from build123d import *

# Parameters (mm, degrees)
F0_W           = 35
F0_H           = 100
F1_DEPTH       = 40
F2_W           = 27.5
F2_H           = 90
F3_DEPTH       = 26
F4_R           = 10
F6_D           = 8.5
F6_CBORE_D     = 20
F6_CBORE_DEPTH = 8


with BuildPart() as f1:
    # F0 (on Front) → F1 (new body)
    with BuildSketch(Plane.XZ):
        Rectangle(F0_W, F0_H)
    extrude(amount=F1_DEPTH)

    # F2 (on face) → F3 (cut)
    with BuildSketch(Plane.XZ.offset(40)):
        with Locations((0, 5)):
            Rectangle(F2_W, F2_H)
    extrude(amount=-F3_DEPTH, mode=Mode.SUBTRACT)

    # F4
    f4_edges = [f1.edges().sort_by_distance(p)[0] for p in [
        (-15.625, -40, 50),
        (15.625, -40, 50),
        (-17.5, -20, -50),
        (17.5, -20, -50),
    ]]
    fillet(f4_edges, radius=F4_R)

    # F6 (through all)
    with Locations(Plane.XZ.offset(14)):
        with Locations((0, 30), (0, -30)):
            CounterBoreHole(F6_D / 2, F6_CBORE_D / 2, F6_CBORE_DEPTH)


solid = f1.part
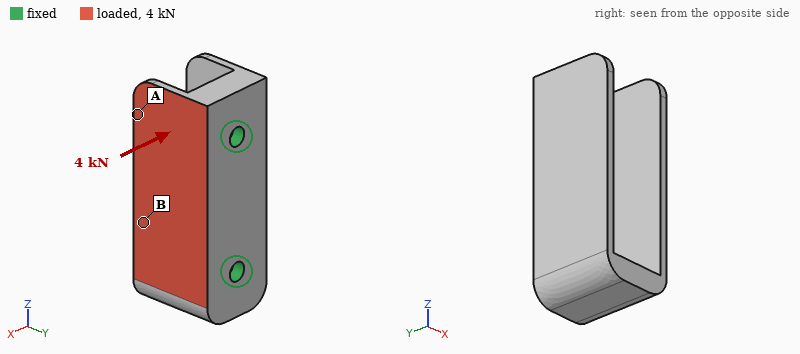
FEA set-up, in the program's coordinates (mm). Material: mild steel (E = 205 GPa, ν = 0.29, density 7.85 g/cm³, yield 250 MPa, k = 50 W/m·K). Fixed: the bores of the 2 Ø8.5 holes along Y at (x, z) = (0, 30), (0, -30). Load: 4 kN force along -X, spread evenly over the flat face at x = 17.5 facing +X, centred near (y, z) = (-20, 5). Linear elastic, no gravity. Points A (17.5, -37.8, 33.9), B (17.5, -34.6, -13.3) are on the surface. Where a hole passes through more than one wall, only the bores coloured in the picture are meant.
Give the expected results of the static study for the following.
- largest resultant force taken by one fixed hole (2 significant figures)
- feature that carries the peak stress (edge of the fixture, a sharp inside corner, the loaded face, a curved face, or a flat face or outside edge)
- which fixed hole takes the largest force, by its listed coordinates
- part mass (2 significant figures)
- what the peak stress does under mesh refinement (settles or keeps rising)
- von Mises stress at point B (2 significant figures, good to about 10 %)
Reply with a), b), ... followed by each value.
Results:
a) 2.3 kN
b) edge of the fixture
c) (0, 30)
d) 530 g
e) keeps rising
f) 47 MPa
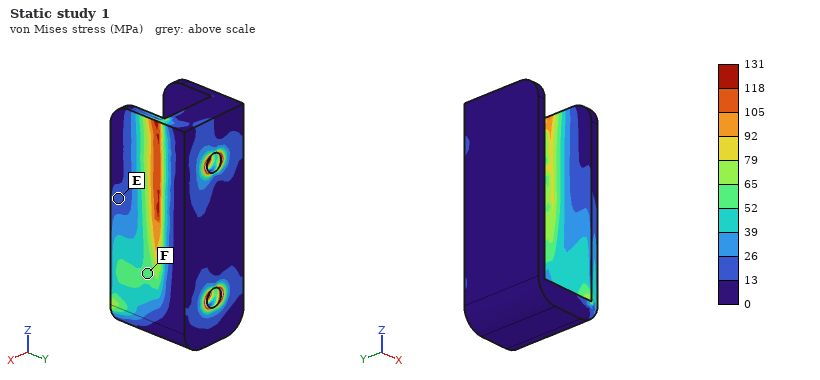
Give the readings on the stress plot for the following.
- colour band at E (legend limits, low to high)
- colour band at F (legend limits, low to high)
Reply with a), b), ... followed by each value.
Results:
a) 13 to 26 MPa
b) 52 to 65 MPa
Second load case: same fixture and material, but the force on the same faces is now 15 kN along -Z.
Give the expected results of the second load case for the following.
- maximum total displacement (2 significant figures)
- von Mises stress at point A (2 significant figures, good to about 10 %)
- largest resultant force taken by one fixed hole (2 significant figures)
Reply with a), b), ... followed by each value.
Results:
a) 29 µm
b) 28 MPa
c) 9.5 kN
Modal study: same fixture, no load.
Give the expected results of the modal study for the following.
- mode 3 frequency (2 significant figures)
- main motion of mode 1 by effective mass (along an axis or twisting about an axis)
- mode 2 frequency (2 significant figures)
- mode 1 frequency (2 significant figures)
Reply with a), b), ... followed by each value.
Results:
a) 4400 Hz
b) along X
c) 4300 Hz
d) 3100 Hz
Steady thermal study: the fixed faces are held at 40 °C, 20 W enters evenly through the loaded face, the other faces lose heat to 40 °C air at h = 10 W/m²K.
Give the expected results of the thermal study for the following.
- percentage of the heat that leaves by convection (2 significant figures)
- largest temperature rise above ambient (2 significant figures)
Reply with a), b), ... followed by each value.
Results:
a) 6.9 %
b) 21 K
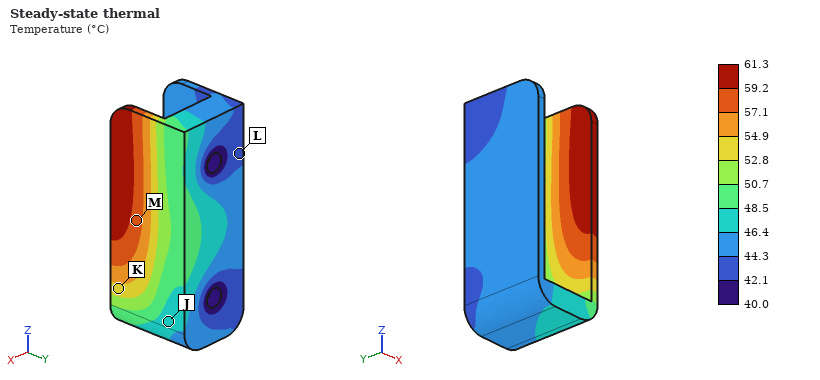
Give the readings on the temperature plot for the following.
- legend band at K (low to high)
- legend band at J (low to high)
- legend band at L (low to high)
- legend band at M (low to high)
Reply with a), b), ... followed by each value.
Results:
a) 52.8 to 54.9 °C
b) 46.4 to 48.5 °C
c) 42.1 to 44.3 °C
d) 57.1 to 59.2 °C
